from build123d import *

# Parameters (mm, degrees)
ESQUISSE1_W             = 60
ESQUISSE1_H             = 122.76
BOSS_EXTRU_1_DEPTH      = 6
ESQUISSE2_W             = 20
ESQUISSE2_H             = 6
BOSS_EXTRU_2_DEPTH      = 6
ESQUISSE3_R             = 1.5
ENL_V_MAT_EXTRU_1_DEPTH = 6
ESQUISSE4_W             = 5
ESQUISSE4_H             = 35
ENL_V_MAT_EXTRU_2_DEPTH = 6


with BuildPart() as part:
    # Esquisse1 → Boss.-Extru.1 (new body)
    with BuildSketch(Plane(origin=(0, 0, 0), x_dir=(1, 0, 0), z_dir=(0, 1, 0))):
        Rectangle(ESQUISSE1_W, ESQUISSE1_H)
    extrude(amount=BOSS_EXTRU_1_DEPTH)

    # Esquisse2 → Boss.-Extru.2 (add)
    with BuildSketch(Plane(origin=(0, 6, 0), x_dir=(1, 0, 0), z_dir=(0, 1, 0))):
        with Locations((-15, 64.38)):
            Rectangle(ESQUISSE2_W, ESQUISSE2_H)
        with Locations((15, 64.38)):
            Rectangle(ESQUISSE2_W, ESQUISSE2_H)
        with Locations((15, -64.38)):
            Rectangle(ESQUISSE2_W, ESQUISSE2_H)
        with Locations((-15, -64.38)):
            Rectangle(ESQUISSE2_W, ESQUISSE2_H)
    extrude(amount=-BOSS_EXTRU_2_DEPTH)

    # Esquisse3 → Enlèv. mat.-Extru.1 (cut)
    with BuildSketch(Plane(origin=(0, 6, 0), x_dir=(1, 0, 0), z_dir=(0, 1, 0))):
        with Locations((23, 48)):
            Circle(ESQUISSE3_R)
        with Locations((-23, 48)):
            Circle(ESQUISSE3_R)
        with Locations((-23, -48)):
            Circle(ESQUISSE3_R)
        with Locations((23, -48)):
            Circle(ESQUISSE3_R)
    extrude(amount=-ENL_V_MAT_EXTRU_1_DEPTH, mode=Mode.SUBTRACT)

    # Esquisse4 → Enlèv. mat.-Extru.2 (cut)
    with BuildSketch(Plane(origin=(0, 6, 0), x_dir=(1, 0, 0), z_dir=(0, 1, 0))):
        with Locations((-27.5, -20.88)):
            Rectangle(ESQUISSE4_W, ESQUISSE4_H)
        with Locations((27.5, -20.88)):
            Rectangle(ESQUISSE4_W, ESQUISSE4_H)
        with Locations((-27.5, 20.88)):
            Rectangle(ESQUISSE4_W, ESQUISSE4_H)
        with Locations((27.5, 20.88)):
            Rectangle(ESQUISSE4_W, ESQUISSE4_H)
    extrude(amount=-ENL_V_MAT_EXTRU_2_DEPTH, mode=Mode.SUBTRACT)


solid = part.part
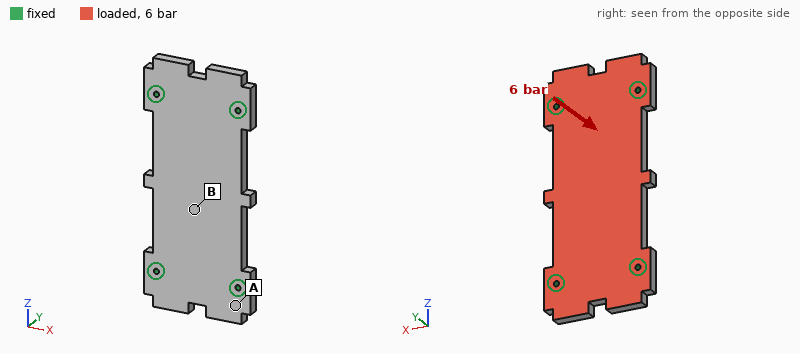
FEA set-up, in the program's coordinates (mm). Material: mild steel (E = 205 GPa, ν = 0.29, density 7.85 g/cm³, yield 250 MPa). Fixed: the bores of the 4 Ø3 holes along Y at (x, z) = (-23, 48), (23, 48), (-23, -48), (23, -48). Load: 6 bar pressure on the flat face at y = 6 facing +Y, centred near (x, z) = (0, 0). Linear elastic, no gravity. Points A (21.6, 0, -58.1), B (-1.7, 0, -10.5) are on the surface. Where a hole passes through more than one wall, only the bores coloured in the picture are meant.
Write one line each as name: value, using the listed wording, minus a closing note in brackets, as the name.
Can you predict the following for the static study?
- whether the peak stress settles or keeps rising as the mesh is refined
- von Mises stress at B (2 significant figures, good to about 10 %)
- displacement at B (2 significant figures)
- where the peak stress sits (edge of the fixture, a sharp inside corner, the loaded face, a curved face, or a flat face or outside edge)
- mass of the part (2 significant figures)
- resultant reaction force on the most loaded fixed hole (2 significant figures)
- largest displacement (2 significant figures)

whether the peak stress settles or keeps rising as the mesh is refined: keeps rising
von Mises stress at B: 33 MPa
displacement at B: 45 µm
where the peak stress sits: edge of the fixture
mass of the part: 340 g
resultant reaction force on the most loaded fixed hole: 1.1 kN
largest displacement: 52 µm
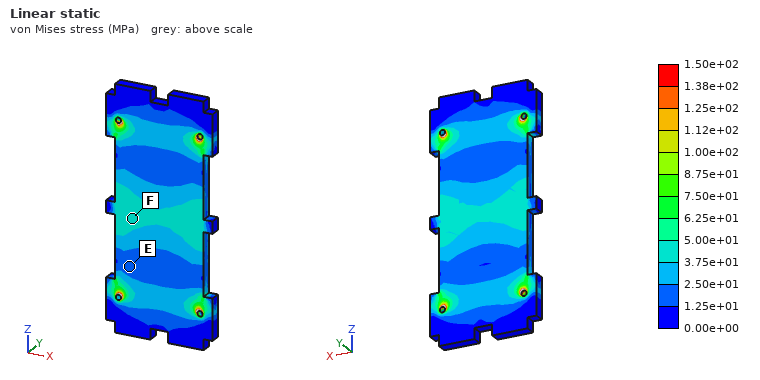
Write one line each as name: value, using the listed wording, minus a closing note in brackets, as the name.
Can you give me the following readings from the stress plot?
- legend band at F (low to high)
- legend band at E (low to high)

legend band at F: 3.75e+01 to 5.00e+01 MPa
legend band at E: 1.25e+01 to 2.50e+01 MPa
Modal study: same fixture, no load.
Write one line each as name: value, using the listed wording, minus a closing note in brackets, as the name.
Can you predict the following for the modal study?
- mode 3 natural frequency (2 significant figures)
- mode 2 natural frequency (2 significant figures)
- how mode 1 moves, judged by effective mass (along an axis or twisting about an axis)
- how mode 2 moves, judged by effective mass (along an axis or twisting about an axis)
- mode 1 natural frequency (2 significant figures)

mode 3 natural frequency: 7500 Hz
mode 2 natural frequency: 5000 Hz
how mode 1 moves, judged by effective mass: along Y
how mode 2 moves, judged by effective mass: twisting about Z
mode 1 natural frequency: 2800 Hz
